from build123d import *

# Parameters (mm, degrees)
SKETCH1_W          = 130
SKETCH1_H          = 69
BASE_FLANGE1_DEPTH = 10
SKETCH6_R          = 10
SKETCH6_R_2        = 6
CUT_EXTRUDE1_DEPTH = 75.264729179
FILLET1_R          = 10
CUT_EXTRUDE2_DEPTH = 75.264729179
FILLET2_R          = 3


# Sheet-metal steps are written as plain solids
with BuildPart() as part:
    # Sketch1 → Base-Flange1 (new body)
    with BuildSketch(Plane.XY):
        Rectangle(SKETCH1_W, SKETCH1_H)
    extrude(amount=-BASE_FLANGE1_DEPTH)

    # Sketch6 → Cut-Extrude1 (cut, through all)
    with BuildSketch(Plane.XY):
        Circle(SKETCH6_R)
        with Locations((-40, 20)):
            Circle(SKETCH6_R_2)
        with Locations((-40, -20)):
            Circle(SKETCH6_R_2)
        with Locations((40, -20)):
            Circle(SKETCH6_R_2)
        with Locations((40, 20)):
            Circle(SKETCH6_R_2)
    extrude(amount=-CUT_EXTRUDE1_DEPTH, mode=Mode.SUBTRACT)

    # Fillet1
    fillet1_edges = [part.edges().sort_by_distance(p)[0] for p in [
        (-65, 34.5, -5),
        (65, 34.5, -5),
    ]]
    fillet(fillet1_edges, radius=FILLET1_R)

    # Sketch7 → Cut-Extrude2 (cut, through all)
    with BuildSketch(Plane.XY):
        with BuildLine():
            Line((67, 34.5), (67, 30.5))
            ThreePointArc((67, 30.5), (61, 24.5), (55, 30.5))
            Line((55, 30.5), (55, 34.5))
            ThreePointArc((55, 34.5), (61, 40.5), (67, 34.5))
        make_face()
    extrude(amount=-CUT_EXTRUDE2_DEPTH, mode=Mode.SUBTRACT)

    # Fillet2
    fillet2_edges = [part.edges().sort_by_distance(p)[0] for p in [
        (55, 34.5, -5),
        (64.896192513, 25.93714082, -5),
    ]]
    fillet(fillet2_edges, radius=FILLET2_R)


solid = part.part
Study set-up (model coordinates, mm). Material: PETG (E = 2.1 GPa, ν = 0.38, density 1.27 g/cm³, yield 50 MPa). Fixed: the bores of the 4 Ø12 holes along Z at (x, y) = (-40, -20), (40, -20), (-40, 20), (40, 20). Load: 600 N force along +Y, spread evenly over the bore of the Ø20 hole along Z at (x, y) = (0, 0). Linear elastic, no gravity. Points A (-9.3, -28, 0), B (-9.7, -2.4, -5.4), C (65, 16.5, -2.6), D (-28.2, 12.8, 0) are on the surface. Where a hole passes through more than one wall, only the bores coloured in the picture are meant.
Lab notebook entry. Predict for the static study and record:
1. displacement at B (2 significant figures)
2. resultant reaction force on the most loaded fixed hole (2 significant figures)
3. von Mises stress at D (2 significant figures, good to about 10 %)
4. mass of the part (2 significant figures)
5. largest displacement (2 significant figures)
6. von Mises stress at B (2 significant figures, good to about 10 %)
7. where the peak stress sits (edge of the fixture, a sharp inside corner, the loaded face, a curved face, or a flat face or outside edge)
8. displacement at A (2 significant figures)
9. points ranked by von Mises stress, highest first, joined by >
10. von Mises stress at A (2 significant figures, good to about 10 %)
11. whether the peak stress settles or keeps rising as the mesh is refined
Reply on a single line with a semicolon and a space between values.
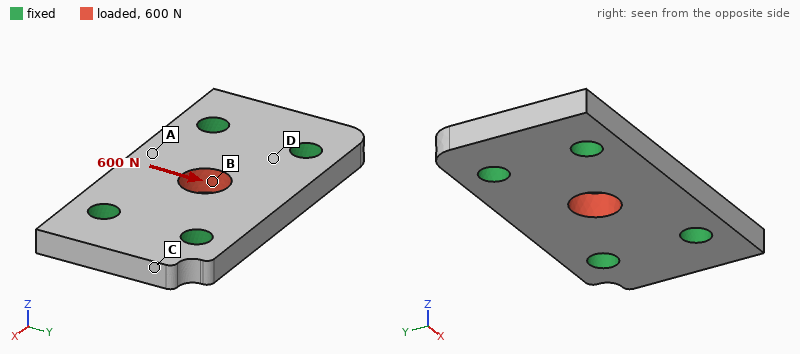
22 µm; 180 N; 1.0 MPa; 100 g; 26 µm; 1.7 MPa; edge of the fixture; 19 µm; B > D > A > C; 0.54 MPa; keeps rising
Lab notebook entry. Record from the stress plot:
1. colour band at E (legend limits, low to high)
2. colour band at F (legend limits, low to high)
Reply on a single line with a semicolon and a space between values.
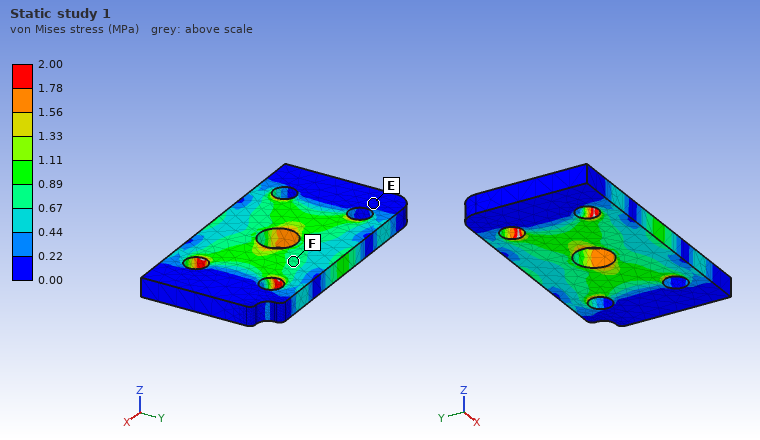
0.00 to 0.22 MPa; 0.67 to 0.89 MPa
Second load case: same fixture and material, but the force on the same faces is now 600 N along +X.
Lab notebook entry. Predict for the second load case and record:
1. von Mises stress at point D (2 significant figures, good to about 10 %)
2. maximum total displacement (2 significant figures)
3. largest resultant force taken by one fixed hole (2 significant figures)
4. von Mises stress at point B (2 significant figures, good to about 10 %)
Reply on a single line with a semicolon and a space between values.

0.73 MPa; 12 µm; 160 N; 0.89 MPa
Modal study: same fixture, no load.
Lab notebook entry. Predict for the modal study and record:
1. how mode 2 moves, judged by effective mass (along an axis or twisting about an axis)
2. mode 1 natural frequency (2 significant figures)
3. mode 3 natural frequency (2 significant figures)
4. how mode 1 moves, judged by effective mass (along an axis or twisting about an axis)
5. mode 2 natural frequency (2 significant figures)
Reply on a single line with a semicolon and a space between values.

twisting about X; 2200 Hz; 3700 Hz; along Z; 2600 Hz
